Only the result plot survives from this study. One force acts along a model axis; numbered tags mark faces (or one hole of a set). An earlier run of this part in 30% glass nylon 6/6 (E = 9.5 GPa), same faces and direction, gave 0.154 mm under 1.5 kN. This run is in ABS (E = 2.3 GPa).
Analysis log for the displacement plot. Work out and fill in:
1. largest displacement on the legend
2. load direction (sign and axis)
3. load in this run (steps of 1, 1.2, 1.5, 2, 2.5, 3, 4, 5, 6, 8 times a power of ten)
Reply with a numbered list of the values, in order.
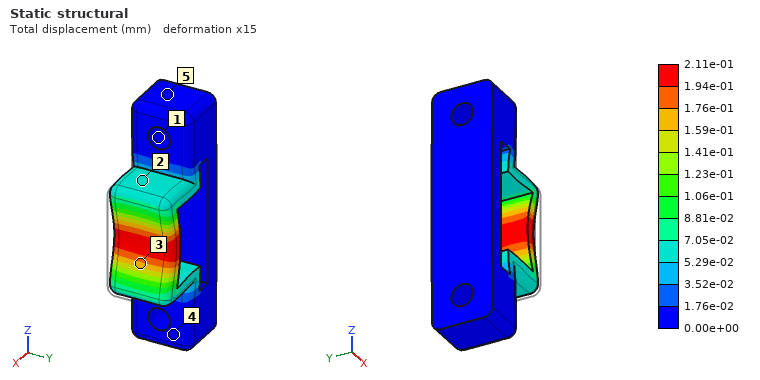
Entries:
1. 2.11e-01 mm
2. -X
3. 500 N
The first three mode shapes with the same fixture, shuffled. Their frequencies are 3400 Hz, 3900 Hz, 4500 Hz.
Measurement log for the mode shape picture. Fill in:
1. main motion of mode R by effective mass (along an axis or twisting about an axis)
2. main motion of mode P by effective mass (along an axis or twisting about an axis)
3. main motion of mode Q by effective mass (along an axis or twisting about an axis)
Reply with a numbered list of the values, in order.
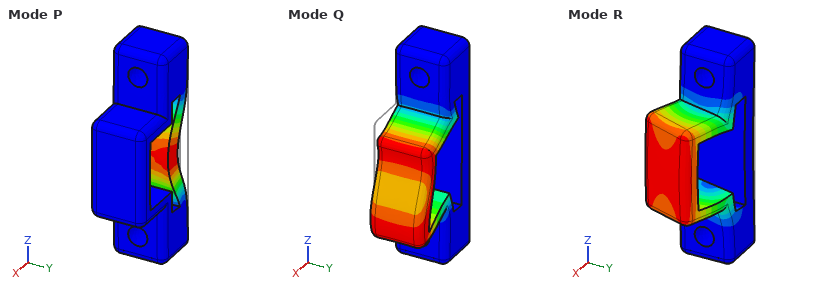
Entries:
1. along Y
2. along X
3. along Z
